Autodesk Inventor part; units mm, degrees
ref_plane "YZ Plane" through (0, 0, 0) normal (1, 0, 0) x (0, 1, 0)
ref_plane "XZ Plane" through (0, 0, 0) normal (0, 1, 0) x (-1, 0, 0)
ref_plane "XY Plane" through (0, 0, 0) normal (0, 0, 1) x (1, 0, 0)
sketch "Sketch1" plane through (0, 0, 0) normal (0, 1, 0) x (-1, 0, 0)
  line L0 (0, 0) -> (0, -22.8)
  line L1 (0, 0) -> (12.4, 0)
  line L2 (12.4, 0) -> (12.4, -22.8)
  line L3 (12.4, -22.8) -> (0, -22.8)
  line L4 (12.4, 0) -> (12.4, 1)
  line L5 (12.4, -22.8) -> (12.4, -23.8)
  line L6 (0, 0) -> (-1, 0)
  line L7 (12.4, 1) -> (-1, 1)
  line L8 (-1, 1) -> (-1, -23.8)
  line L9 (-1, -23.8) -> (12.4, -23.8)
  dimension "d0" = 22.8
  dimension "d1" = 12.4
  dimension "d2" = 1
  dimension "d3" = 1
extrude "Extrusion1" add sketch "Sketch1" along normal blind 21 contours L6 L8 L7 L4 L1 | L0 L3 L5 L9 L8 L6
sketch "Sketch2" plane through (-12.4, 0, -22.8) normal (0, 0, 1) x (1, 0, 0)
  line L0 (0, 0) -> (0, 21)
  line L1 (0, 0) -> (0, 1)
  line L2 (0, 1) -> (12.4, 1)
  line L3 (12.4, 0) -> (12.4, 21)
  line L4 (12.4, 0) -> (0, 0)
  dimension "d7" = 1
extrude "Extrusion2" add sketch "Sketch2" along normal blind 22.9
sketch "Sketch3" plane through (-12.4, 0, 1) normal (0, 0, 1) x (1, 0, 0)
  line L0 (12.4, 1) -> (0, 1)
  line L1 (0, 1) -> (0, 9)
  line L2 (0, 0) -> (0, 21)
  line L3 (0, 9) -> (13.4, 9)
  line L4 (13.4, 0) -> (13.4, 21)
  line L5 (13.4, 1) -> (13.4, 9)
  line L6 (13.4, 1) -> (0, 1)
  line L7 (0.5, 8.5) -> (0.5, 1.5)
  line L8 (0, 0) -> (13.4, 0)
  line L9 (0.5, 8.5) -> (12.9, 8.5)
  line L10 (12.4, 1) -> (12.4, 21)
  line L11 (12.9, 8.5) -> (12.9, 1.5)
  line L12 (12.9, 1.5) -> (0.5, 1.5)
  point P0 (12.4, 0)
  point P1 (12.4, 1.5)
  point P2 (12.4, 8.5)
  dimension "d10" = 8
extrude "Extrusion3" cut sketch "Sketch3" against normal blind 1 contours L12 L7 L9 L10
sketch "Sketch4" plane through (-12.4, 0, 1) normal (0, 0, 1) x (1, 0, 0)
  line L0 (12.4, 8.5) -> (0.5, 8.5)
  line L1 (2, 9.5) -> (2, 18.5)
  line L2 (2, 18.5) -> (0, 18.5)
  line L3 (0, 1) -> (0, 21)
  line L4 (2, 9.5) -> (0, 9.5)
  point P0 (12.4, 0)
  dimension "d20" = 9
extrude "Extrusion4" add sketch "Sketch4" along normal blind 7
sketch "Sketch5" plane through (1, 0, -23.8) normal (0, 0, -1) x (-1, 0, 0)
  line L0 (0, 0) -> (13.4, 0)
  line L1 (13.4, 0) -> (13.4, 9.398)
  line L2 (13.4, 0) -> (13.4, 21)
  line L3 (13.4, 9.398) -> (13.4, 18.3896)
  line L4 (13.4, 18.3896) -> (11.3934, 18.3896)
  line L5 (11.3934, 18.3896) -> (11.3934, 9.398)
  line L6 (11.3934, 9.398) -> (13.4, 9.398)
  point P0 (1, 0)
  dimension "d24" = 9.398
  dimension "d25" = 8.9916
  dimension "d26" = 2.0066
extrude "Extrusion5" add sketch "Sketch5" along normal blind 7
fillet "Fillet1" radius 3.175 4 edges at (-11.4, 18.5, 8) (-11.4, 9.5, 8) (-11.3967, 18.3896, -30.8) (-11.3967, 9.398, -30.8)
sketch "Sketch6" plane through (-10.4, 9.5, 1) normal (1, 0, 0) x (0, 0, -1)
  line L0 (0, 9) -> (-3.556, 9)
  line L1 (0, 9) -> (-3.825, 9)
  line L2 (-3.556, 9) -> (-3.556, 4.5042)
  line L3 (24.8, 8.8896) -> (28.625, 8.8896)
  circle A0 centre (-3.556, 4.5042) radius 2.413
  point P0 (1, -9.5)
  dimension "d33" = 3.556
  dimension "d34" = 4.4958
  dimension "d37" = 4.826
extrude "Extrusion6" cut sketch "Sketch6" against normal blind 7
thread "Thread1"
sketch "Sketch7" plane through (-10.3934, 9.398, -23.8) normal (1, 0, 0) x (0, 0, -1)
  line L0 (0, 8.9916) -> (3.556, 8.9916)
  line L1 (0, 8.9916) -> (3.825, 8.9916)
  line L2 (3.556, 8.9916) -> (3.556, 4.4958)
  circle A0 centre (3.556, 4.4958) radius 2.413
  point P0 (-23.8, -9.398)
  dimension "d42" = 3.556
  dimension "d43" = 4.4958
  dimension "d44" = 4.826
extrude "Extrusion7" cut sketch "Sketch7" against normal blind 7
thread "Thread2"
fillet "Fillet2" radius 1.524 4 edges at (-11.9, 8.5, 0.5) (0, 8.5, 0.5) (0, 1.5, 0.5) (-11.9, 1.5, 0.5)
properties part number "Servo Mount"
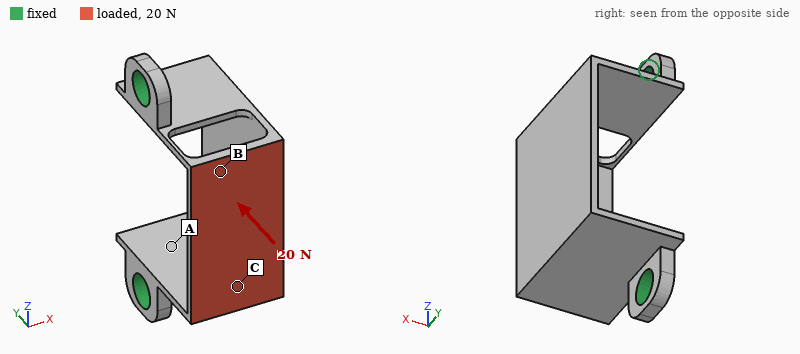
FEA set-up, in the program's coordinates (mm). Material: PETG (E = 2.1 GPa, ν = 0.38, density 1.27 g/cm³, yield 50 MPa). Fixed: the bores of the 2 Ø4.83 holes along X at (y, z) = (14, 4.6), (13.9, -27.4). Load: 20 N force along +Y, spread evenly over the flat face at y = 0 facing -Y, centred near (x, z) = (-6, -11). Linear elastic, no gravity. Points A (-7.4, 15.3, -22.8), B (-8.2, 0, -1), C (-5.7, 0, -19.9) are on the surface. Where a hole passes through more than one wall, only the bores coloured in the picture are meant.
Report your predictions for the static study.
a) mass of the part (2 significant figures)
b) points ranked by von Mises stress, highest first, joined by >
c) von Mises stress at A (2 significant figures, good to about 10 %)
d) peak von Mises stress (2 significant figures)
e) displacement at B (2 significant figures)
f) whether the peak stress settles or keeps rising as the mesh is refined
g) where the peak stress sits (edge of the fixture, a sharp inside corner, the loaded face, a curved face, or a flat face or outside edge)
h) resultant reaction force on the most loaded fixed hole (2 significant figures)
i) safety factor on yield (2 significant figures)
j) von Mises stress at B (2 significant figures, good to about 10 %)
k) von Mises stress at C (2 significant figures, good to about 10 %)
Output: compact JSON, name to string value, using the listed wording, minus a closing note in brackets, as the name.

{"mass of the part": "1.8 g", "points ranked by von Mises stress, highest first, joined by >": "B > C > A", "von Mises stress at A": "1.5 MPa", "peak von Mises stress": "42 MPa", "displacement at B": "0.15 mm", "whether the peak stress settles or keeps rising as the mesh is refined": "settles", "where the peak stress sits": "a curved face", "resultant reaction force on the most loaded fixed hole": "10 N", "safety factor on yield": "1.2", "von Mises stress at B": "7.7 MPa", "von Mises stress at C": "5.3 MPa"}
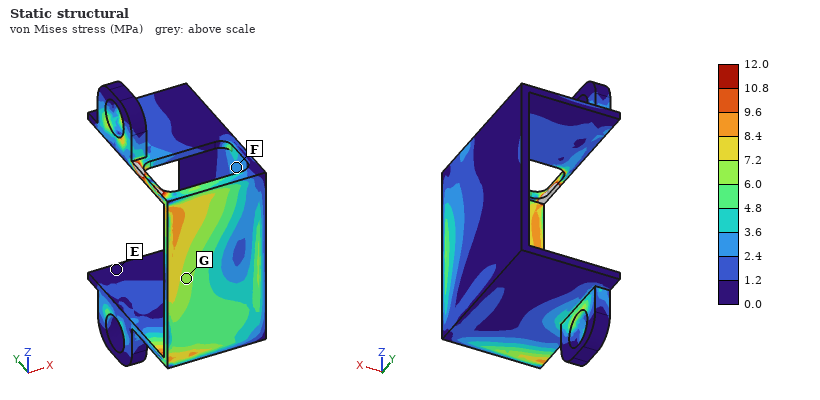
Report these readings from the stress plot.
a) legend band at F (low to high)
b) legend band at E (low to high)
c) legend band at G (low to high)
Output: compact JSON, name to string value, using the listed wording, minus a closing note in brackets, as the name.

{"legend band at F": "2.4 to 3.6 MPa", "legend band at E": "0.0 to 1.2 MPa", "legend band at G": "6.0 to 7.2 MPa"}
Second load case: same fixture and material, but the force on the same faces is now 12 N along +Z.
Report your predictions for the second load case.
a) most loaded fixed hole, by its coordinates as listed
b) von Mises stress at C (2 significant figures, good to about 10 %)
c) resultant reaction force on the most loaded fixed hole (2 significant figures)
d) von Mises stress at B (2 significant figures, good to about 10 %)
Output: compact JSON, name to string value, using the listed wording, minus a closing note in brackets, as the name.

{"most loaded fixed hole, by its coordinates as listed": "(13.9, -27.4)", "von Mises stress at C": "3.3 MPa", "resultant reaction force on the most loaded fixed hole": "9.4 N", "von Mises stress at B": "2.1 MPa"}
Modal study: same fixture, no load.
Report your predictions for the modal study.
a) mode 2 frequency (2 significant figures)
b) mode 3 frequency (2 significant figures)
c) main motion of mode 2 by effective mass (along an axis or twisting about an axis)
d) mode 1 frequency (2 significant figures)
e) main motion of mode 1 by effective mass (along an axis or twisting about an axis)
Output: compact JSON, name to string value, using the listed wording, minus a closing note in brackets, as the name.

{"mode 2 frequency": "1100 Hz", "mode 3 frequency": "1500 Hz", "main motion of mode 2 by effective mass": "along X", "mode 1 frequency": "860 Hz", "main motion of mode 1 by effective mass": "along Z"}
